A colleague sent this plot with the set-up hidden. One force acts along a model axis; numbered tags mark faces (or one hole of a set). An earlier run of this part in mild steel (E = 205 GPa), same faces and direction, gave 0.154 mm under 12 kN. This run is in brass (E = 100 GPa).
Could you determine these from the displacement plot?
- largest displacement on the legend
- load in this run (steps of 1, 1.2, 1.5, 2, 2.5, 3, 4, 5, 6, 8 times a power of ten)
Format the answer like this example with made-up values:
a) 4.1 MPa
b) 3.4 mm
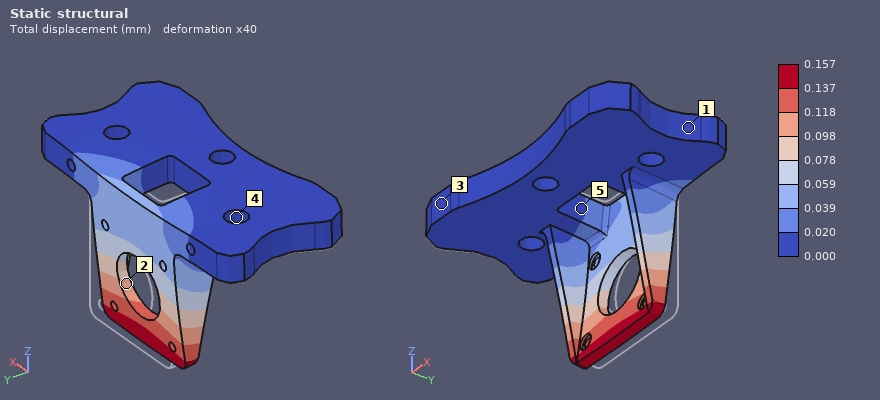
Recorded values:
a) 0.157 mm
b) 6 kN
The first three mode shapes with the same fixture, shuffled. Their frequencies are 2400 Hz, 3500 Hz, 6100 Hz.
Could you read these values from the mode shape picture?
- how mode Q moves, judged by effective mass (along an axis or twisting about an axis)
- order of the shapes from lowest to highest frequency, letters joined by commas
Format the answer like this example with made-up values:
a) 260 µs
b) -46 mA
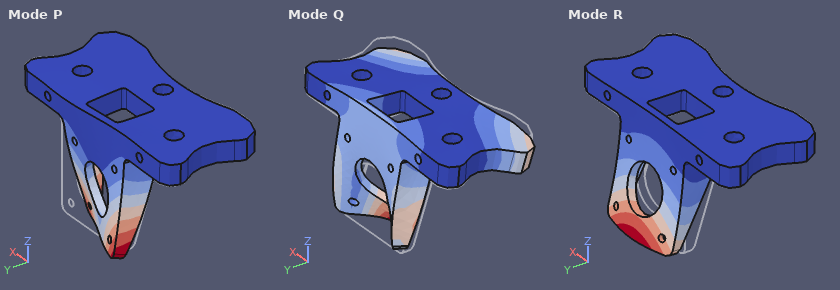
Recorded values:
a) twisting about X
b) R, P, Q
